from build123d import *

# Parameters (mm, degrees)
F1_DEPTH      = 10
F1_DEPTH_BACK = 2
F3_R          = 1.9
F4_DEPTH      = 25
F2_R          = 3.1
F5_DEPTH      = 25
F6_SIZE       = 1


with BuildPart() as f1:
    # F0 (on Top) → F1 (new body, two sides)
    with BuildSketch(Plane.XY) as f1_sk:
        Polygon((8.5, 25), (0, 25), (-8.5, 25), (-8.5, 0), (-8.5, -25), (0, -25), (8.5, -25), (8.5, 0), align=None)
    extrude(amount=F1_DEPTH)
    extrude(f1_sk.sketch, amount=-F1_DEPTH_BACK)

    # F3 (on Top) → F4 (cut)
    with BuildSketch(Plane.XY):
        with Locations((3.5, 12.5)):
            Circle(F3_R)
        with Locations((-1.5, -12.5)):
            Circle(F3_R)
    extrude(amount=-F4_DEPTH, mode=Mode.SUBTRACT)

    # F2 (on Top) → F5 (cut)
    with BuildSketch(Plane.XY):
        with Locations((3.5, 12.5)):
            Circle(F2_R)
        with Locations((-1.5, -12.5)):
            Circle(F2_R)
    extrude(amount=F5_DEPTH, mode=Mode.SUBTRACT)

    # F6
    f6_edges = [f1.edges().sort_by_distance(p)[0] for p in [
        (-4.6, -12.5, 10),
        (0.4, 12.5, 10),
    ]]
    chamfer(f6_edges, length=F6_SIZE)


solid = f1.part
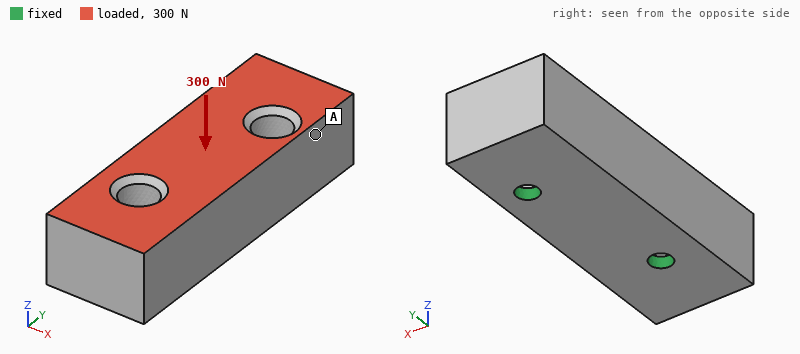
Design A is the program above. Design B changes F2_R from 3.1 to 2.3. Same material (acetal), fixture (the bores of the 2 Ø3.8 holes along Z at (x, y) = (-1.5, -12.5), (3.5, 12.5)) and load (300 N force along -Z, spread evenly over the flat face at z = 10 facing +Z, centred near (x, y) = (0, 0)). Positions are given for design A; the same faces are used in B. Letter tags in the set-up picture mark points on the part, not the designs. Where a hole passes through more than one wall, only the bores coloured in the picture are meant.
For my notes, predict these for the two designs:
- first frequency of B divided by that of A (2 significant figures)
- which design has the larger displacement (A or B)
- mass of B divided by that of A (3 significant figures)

1.1
A
1.03
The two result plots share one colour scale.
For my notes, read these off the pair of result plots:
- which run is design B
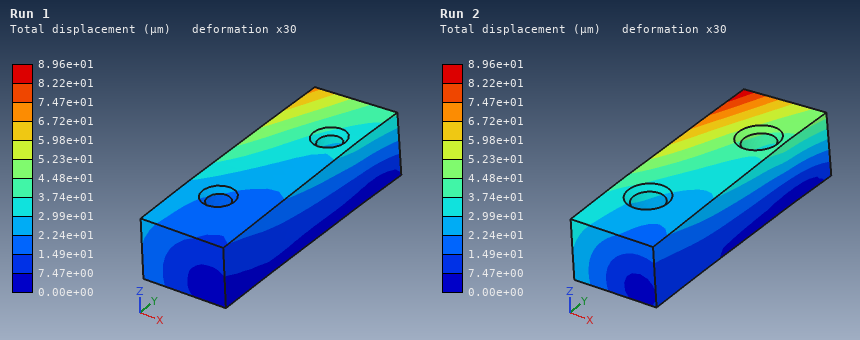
Run 1
